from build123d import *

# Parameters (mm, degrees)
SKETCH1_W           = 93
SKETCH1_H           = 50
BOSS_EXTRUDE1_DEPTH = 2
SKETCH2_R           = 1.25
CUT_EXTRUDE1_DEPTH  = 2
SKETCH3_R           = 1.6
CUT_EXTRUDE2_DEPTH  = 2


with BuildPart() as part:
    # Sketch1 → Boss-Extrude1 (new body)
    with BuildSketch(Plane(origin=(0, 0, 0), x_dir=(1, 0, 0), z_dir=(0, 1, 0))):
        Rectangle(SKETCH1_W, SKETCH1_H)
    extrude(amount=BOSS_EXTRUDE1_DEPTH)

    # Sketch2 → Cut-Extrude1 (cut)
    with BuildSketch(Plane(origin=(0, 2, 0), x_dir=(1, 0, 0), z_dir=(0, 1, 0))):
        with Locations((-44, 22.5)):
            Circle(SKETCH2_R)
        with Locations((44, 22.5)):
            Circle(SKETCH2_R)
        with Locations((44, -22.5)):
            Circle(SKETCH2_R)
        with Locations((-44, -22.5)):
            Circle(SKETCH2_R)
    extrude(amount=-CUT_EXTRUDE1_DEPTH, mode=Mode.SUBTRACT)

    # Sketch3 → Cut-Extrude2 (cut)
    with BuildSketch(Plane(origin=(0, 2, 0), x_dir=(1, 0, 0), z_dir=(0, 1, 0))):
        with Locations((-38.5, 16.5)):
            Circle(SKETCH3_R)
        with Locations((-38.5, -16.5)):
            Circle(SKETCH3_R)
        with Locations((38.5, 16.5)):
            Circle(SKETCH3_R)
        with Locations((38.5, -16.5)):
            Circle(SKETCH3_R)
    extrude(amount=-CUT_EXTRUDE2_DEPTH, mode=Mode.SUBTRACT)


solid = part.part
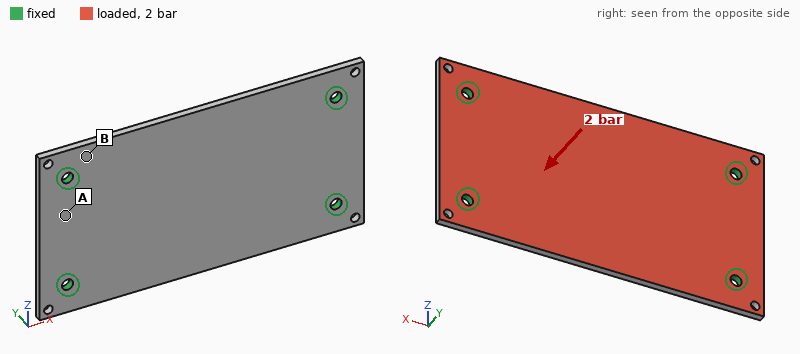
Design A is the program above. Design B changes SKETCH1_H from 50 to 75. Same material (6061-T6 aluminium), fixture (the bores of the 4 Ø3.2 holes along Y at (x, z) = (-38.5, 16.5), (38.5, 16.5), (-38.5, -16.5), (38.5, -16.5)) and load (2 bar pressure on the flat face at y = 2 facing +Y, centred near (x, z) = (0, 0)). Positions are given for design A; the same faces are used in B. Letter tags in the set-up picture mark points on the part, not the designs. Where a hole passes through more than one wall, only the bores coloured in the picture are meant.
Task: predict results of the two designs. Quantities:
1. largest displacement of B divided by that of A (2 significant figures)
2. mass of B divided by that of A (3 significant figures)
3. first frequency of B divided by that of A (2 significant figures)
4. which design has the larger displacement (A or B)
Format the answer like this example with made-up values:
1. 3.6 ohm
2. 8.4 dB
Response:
1. 1.5
2. 1.51
3. 0.90
4. B
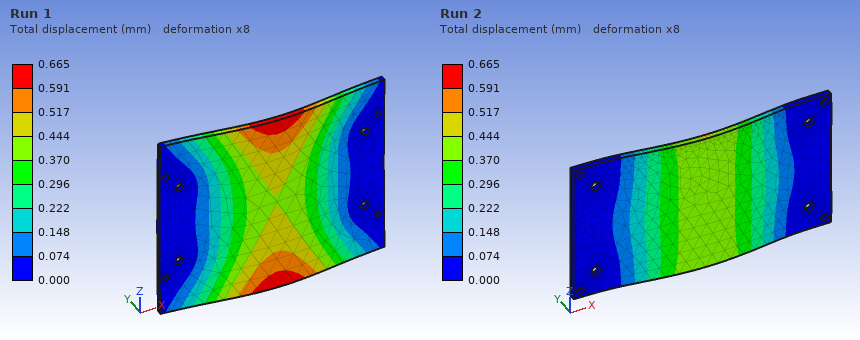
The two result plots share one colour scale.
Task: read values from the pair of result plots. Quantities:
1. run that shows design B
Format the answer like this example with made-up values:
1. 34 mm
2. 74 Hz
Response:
1. Run 1
